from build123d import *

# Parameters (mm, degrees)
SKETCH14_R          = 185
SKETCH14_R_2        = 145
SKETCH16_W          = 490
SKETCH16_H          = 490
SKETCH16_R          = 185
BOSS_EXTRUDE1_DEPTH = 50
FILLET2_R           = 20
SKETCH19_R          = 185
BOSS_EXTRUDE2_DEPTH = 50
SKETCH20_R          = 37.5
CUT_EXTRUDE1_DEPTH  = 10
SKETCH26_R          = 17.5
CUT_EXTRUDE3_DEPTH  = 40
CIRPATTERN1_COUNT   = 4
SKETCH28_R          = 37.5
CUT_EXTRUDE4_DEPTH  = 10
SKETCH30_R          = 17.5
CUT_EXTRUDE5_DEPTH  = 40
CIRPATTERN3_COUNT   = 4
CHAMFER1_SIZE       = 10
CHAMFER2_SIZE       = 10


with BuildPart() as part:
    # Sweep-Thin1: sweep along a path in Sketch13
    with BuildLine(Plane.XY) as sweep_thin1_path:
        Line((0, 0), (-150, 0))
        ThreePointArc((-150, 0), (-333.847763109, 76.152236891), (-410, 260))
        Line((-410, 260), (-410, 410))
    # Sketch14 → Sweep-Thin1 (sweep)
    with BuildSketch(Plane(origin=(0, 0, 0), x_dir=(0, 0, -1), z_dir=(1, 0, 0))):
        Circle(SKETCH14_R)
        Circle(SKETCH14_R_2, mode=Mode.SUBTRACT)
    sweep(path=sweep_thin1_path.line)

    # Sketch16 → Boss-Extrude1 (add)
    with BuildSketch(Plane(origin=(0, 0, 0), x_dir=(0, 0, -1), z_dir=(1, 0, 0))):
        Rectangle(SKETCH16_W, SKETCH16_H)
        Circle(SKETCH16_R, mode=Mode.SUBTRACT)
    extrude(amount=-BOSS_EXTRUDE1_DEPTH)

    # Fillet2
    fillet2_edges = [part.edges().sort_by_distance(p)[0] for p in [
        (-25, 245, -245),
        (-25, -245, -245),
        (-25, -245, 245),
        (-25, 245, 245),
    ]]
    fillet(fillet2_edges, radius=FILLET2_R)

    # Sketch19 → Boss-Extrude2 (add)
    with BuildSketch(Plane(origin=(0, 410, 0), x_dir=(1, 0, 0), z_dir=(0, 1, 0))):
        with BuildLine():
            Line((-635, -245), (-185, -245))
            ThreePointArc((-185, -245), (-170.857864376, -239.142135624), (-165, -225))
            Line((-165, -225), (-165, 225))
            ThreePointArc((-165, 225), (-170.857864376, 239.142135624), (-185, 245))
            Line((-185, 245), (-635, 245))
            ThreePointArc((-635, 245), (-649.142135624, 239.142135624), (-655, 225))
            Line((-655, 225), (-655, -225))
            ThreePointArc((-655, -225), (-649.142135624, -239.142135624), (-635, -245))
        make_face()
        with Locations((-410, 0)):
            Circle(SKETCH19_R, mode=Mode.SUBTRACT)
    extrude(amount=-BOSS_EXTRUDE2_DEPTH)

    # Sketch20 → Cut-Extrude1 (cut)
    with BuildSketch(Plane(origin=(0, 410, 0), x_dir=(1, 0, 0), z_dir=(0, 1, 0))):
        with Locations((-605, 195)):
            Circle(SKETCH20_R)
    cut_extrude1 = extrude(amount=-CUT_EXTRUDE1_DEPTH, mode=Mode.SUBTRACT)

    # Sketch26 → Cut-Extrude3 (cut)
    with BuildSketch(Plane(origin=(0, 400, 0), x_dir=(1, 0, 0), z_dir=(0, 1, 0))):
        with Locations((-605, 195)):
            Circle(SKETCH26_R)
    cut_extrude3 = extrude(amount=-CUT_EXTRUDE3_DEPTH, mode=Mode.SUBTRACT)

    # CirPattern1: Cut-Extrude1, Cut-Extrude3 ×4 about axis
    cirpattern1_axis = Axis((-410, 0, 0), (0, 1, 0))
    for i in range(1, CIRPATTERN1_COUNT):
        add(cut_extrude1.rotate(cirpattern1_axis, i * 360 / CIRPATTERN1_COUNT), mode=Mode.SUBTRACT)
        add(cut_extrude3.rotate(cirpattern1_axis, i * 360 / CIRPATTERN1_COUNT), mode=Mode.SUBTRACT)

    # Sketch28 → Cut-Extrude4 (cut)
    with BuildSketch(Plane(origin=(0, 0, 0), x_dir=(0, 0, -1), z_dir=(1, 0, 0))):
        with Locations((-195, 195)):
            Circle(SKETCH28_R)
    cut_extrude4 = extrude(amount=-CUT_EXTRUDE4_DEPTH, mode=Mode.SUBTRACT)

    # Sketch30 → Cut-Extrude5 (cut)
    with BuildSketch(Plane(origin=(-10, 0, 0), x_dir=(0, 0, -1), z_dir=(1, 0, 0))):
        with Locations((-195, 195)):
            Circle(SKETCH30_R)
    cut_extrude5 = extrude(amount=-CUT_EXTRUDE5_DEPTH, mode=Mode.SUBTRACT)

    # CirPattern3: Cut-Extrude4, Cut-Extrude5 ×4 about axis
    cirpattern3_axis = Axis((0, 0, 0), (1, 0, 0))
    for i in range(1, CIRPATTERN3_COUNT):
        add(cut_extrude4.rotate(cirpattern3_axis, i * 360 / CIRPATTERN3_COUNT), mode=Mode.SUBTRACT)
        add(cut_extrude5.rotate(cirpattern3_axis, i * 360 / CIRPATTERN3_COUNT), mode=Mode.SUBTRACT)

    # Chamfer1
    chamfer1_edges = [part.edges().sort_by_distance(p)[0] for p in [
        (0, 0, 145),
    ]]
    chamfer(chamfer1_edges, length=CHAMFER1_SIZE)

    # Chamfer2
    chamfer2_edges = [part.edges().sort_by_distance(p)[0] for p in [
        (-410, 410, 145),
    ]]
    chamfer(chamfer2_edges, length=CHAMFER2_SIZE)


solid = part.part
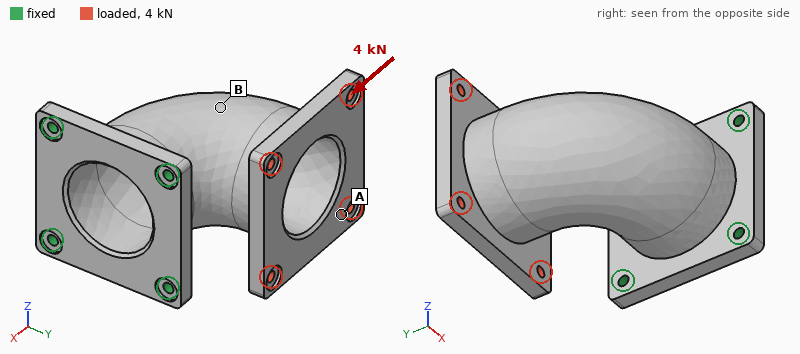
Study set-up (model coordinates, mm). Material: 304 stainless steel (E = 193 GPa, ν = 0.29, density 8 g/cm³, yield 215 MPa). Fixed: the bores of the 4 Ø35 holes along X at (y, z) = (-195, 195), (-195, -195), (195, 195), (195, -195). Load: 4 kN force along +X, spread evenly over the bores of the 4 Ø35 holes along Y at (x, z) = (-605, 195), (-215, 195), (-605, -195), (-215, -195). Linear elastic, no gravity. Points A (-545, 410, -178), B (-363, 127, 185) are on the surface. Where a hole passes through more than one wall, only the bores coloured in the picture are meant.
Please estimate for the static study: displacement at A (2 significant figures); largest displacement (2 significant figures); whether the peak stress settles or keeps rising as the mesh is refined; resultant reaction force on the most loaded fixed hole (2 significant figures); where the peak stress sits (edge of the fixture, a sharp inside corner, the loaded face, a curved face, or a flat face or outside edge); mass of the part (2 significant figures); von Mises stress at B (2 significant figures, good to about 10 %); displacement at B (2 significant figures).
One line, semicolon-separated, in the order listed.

16 µm; 18 µm; keeps rising; 3.2 kN; edge of the fixture; 330 kg; 0.44 MPa; 6.8 µm
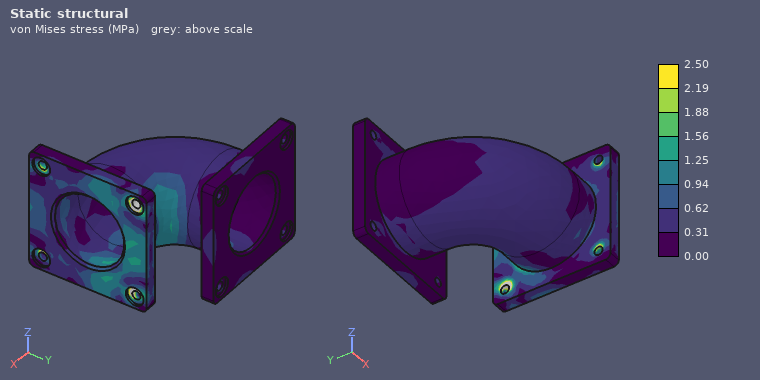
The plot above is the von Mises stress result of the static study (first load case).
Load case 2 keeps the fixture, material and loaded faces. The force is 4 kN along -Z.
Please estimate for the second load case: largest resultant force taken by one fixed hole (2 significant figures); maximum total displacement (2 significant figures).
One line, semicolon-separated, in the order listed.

2.9 kN; 17 µm
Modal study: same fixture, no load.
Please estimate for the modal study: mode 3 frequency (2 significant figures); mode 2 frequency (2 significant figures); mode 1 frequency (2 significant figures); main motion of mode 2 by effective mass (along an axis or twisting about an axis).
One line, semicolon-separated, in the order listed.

560 Hz; 230 Hz; 200 Hz; along Z
